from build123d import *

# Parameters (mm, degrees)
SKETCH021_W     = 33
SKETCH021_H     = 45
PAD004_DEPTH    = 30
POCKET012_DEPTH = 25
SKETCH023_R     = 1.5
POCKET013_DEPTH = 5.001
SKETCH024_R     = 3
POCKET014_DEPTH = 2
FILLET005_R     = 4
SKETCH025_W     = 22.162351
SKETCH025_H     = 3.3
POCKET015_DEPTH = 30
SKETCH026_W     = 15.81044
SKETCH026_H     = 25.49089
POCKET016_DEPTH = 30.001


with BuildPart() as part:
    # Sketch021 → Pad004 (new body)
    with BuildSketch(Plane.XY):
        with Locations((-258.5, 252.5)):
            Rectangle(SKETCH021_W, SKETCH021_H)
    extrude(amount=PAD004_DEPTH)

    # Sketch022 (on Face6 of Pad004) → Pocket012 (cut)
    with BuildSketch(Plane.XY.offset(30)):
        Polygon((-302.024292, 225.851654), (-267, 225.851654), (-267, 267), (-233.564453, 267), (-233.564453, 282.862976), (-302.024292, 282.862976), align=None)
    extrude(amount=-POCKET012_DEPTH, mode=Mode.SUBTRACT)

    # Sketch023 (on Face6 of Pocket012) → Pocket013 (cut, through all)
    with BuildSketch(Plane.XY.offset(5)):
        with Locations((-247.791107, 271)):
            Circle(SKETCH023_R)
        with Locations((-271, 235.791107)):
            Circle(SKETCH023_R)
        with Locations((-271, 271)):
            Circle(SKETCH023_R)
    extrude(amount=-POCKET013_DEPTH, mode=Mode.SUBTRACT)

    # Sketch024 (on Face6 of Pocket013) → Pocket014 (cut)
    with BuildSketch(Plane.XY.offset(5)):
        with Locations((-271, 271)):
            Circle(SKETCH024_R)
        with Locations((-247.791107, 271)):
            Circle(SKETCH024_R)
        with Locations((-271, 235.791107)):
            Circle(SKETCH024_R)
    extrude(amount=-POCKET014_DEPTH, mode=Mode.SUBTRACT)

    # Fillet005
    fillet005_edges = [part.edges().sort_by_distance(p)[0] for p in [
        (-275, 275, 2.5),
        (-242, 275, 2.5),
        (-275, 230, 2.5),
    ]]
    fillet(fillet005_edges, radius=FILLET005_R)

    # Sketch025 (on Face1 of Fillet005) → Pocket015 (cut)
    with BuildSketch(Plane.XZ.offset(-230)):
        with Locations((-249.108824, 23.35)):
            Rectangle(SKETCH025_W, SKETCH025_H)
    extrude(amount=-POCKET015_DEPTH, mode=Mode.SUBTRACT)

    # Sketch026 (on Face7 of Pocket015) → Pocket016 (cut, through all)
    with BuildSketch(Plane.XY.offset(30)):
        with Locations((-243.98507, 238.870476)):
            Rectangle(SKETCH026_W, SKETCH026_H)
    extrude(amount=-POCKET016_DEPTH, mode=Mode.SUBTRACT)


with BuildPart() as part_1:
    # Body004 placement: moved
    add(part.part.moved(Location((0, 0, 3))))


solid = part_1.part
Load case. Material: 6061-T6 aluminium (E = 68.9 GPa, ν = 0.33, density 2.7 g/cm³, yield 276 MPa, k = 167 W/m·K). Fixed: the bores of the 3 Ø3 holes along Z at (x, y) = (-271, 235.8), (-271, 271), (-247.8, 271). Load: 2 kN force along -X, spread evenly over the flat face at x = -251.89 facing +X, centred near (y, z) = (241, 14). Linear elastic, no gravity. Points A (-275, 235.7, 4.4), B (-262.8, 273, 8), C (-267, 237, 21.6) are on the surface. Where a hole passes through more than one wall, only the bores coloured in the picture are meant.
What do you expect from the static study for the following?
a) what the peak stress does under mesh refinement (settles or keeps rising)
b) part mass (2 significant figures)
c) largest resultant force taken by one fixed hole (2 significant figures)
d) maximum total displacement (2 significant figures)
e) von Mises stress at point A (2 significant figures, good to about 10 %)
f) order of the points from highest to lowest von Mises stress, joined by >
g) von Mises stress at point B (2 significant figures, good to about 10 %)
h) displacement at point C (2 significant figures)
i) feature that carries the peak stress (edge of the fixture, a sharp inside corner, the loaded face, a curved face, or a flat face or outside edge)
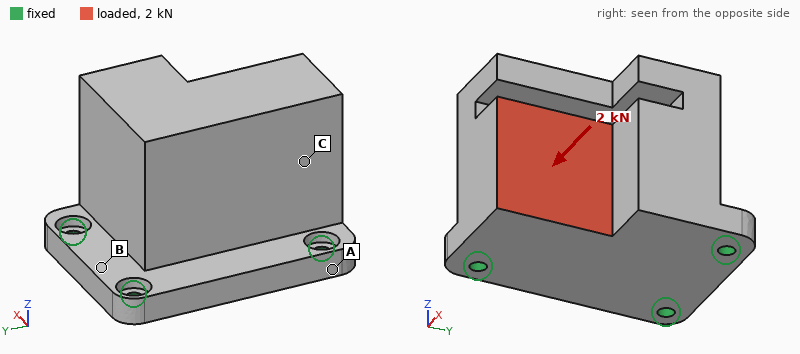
keeps rising
61 g
1.2 kN
52 µm
32 MPa
A > B > C
19 MPa
30 µm
edge of the fixture
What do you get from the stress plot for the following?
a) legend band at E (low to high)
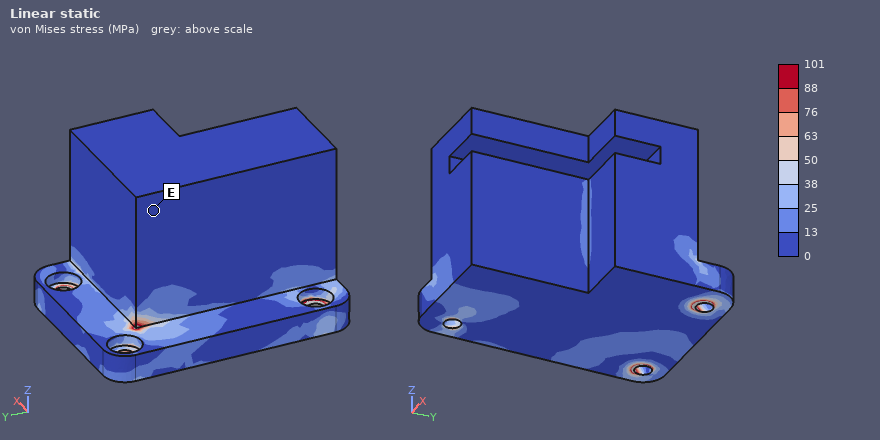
0 to 13 MPa
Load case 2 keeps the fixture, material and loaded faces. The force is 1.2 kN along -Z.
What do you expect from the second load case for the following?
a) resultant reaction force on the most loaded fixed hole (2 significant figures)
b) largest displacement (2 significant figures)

1.1 kN
59 µm
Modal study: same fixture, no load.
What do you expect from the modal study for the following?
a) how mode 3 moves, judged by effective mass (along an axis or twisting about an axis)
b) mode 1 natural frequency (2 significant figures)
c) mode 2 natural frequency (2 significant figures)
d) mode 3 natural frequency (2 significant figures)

along Z
4300 Hz
9300 Hz
11 kHz
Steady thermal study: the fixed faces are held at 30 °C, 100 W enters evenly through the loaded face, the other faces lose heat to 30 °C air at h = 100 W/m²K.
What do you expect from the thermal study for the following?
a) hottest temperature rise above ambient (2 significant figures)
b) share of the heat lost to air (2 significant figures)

47 K
17 %
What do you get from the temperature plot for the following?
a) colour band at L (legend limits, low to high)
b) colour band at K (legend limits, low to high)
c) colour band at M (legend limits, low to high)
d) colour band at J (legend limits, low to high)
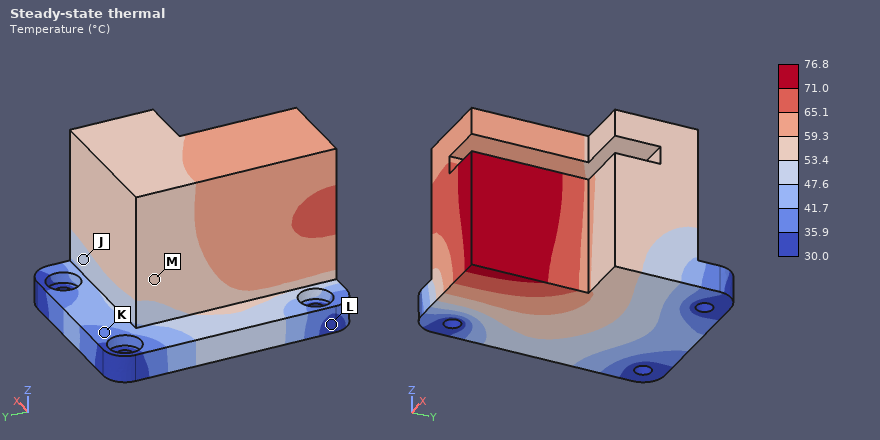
30.0 to 35.9 °C
35.9 to 41.7 °C
53.4 to 59.3 °C
47.6 to 53.4 °C
